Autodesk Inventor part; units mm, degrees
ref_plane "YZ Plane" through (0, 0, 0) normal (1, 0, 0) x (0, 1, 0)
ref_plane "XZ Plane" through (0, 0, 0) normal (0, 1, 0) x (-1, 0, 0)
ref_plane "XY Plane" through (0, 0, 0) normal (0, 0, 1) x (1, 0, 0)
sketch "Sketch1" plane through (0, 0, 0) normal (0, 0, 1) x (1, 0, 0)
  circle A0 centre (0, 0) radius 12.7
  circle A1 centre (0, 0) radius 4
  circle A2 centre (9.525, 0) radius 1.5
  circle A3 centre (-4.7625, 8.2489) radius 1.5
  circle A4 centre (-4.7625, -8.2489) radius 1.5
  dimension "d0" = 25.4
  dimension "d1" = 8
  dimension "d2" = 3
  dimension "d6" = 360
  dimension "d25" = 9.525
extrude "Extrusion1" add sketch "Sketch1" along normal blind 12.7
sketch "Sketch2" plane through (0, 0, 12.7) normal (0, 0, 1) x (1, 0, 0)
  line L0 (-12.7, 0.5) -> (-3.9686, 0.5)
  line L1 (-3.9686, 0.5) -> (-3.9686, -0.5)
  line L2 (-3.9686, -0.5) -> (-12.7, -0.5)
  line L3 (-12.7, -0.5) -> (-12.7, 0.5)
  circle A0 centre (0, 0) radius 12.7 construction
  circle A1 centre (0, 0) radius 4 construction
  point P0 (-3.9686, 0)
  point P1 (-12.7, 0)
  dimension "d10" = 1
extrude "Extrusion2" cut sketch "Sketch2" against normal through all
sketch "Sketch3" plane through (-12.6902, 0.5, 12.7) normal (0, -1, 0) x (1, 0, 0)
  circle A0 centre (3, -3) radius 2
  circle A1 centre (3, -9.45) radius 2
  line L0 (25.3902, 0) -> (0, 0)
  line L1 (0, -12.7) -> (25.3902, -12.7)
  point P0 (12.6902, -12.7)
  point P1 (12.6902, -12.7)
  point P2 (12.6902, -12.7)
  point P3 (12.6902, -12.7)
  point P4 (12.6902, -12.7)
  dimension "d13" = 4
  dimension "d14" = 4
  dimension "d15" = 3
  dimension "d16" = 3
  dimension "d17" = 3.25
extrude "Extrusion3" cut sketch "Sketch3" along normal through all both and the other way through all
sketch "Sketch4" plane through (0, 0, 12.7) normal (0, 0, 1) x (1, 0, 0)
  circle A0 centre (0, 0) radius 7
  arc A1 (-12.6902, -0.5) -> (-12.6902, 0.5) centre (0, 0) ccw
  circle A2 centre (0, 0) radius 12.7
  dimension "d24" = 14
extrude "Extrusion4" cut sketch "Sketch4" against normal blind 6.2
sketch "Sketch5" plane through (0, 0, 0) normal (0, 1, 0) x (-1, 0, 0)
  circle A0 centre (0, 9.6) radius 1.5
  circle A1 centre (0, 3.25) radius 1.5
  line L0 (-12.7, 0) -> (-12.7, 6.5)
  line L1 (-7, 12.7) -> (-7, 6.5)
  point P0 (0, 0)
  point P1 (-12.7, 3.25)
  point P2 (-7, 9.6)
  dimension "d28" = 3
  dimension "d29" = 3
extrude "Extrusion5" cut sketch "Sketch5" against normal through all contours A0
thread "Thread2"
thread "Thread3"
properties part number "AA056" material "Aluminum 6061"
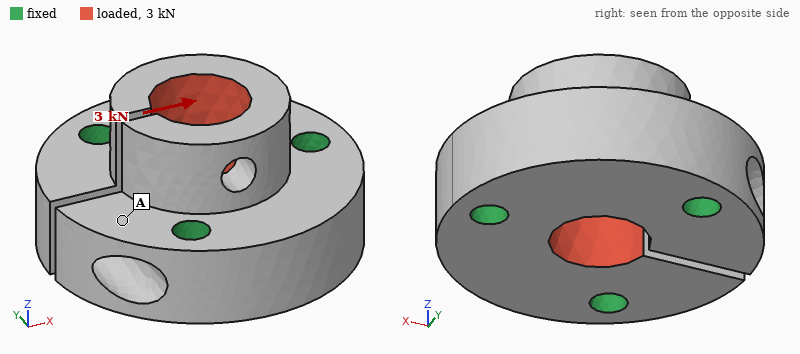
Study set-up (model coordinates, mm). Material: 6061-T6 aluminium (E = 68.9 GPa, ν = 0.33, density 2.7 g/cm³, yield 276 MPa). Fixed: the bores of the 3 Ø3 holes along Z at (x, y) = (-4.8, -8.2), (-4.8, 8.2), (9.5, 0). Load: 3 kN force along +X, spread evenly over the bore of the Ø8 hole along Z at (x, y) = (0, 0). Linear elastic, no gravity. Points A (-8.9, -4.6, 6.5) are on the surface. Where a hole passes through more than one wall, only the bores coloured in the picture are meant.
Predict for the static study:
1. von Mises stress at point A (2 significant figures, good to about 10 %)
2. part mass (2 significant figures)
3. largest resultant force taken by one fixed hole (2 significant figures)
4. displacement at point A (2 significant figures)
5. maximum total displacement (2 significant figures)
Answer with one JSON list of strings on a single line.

["13 MPa", "8.6 g", "1.2 kN", "4.2 µm", "19 µm"]
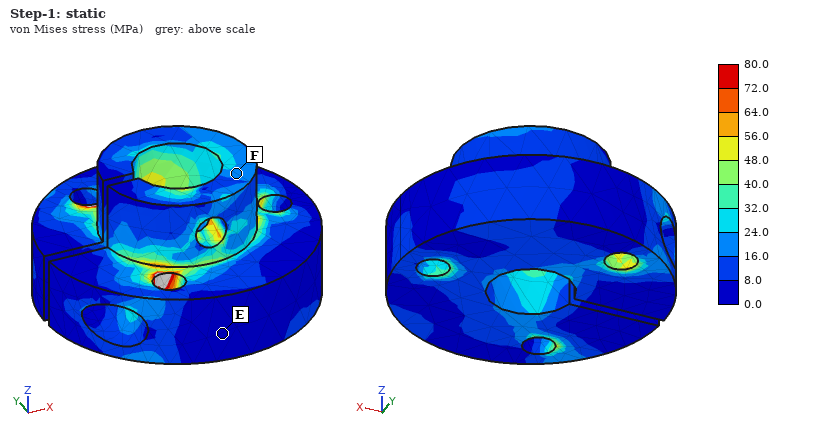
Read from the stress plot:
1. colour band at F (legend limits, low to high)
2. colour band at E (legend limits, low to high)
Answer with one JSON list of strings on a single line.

["16.0 to 24.0 MPa", "0.0 to 8.0 MPa"]
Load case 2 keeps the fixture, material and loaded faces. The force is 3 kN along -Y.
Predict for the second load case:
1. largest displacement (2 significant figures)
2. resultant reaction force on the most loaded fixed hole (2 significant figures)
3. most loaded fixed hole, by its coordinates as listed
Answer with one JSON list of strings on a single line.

["17 µm", "1.2 kN", "(9.5, 0)"]
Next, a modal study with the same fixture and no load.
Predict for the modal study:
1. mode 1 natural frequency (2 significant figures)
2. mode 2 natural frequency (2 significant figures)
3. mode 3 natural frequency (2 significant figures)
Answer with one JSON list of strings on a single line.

["39 kHz", "42 kHz", "47 kHz"]
